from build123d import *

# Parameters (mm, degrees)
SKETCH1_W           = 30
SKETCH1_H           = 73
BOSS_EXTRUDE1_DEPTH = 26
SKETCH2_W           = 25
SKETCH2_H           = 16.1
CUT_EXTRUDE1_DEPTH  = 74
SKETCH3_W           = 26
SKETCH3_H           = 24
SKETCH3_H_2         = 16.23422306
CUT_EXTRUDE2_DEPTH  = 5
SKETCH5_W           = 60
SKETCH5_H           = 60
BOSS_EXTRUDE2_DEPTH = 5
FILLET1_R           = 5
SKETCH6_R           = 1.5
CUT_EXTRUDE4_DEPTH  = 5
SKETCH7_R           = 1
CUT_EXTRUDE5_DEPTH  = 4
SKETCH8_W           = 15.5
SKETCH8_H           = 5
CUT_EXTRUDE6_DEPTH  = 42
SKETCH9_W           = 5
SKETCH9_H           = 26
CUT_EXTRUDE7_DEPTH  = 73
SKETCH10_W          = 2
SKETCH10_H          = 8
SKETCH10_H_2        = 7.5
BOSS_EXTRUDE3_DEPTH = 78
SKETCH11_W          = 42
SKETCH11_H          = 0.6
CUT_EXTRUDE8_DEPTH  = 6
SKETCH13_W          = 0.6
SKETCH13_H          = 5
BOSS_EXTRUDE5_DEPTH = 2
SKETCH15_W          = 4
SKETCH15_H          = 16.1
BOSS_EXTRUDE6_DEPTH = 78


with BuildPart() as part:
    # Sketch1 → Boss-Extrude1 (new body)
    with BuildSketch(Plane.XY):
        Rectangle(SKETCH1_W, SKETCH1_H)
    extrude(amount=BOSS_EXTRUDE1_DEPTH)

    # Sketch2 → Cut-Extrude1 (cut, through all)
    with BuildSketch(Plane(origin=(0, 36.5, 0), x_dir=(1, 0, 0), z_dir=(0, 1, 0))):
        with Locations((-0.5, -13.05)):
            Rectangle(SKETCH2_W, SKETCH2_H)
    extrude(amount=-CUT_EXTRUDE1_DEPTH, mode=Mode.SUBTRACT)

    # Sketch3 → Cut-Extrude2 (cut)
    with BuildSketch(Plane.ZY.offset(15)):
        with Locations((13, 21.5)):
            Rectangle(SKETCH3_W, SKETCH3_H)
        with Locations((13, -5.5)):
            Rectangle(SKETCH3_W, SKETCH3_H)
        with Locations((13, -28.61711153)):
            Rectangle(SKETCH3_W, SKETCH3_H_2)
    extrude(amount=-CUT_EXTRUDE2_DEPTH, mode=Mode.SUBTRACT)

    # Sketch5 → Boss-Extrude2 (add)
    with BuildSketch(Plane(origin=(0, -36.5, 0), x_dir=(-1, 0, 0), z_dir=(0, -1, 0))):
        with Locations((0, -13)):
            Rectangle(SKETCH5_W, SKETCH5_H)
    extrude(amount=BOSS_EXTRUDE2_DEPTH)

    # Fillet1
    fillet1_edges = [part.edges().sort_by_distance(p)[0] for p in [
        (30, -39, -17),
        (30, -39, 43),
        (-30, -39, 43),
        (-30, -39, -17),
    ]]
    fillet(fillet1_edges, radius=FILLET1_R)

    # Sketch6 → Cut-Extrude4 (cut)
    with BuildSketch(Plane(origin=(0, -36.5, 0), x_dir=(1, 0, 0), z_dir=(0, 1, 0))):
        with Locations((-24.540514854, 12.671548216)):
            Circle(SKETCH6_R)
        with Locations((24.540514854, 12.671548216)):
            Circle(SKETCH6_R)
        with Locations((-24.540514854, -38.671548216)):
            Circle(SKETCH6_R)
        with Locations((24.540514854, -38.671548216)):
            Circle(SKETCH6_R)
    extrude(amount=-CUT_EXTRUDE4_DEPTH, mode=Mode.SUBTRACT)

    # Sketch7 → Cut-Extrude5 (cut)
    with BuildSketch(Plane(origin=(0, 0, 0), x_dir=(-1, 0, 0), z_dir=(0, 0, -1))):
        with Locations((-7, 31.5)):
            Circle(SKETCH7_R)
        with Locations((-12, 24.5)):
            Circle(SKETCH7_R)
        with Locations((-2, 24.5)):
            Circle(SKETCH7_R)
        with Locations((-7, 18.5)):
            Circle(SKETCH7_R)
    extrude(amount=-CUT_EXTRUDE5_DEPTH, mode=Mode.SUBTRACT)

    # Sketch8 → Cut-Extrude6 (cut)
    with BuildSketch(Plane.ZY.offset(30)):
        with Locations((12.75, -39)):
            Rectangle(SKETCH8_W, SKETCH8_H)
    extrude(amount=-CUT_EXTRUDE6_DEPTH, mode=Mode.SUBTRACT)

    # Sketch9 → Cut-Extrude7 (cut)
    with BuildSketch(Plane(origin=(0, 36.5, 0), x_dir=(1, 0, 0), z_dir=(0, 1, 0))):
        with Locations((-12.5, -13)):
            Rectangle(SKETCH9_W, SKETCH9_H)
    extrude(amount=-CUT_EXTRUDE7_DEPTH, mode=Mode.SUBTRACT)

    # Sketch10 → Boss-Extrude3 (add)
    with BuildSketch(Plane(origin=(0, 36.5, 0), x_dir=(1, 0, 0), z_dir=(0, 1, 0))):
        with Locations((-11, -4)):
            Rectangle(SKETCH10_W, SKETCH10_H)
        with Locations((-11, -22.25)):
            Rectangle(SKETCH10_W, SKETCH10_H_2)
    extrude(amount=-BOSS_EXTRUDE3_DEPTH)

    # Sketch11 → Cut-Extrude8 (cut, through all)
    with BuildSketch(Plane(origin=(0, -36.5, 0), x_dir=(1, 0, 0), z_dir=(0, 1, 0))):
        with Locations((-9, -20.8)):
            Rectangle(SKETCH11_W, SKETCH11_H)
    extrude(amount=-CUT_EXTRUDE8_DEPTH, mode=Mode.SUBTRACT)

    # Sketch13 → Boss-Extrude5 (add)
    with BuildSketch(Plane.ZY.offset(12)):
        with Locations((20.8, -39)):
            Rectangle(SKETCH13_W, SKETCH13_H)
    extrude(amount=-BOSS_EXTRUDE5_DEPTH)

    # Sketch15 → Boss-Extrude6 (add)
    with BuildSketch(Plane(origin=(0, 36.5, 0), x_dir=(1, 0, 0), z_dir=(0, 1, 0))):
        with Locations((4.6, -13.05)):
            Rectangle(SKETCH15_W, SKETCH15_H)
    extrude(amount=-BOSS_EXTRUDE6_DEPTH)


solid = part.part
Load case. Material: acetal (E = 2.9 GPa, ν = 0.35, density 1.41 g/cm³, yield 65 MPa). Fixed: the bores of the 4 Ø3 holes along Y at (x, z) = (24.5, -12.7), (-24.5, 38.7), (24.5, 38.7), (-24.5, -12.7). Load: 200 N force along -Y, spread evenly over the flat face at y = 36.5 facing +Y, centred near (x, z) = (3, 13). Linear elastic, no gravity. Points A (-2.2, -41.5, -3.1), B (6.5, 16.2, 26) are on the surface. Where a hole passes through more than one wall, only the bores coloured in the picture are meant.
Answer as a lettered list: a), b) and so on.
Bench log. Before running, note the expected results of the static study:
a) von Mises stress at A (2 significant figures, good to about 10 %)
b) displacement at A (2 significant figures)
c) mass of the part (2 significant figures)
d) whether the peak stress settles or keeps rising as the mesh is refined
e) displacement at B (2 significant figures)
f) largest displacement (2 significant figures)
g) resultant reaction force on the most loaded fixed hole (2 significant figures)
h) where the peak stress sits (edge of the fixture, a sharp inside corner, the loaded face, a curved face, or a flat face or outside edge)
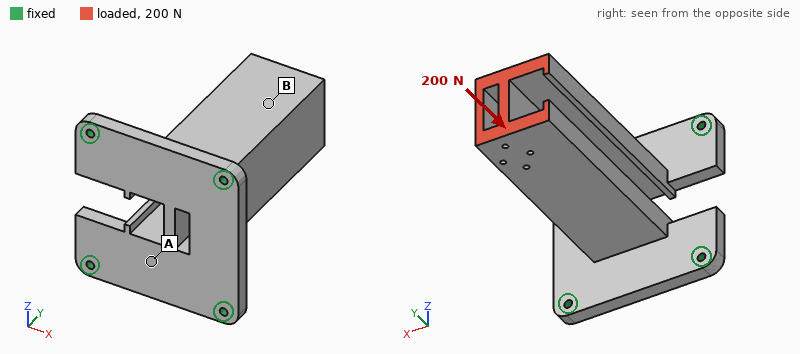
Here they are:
a) 2.5 MPa
b) 0.093 mm
c) 61 g
d) keeps rising
e) 0.12 mm
f) 0.14 mm
g) 60 N
h) edge of the fixture
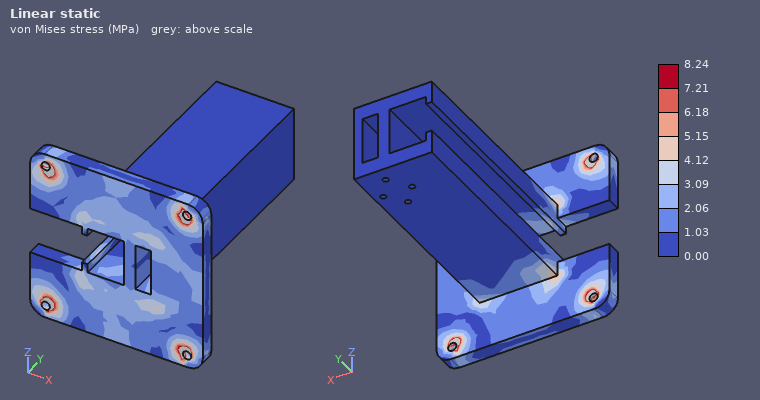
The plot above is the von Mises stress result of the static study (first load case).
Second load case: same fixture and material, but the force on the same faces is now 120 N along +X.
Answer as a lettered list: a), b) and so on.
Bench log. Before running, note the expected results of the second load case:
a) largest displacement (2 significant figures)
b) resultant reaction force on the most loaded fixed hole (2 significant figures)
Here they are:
a) 1.2 mm
b) 110 N
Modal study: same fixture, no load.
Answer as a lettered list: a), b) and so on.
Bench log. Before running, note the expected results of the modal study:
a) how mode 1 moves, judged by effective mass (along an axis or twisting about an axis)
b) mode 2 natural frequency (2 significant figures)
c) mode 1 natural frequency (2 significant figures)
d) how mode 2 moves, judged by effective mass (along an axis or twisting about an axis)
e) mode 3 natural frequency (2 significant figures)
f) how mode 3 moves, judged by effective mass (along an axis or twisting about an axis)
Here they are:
a) along X
b) 460 Hz
c) 430 Hz
d) along Z
e) 1000 Hz
f) along Y
